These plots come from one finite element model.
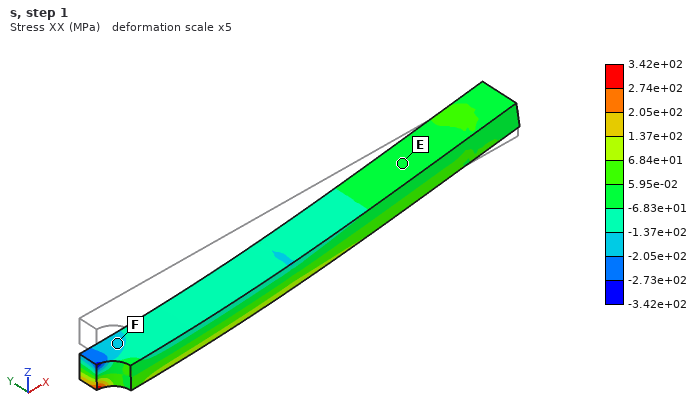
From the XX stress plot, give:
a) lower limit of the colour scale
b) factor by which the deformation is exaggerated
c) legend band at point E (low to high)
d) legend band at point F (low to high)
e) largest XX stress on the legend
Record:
-3.42e+02 MPa
5
-6.83e+01 to 5.95e-02 MPa
-2.05e+02 to -1.37e+02 MPa
3.42e+02 MPa
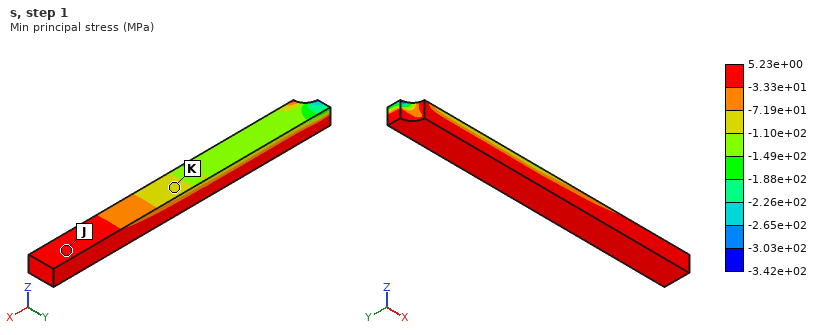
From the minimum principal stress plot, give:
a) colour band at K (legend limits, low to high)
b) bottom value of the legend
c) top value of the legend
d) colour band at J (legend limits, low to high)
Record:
-1.10e+02 to -7.19e+01 MPa
-3.42e+02 MPa
5.23e+00 MPa
-3.33e+01 to 5.23e+00 MPa
